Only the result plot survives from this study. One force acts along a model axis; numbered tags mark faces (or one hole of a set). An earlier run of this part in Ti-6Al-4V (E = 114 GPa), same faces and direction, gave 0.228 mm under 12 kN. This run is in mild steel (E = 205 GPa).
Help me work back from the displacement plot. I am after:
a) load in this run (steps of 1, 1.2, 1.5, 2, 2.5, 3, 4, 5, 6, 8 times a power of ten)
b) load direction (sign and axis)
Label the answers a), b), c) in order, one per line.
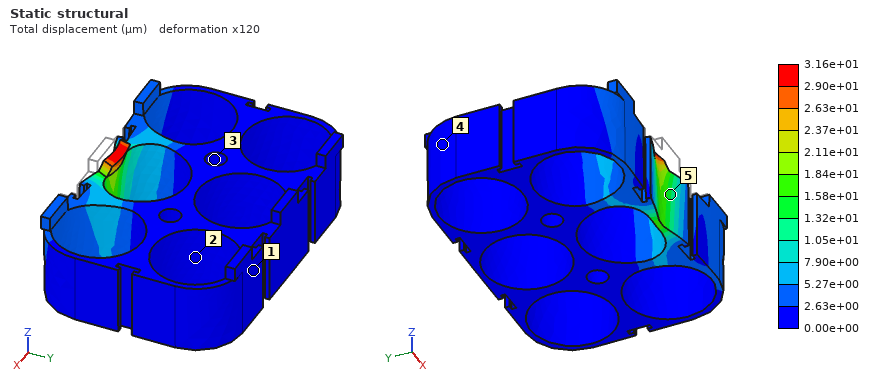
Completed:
a) 3 kN
b) +Y
